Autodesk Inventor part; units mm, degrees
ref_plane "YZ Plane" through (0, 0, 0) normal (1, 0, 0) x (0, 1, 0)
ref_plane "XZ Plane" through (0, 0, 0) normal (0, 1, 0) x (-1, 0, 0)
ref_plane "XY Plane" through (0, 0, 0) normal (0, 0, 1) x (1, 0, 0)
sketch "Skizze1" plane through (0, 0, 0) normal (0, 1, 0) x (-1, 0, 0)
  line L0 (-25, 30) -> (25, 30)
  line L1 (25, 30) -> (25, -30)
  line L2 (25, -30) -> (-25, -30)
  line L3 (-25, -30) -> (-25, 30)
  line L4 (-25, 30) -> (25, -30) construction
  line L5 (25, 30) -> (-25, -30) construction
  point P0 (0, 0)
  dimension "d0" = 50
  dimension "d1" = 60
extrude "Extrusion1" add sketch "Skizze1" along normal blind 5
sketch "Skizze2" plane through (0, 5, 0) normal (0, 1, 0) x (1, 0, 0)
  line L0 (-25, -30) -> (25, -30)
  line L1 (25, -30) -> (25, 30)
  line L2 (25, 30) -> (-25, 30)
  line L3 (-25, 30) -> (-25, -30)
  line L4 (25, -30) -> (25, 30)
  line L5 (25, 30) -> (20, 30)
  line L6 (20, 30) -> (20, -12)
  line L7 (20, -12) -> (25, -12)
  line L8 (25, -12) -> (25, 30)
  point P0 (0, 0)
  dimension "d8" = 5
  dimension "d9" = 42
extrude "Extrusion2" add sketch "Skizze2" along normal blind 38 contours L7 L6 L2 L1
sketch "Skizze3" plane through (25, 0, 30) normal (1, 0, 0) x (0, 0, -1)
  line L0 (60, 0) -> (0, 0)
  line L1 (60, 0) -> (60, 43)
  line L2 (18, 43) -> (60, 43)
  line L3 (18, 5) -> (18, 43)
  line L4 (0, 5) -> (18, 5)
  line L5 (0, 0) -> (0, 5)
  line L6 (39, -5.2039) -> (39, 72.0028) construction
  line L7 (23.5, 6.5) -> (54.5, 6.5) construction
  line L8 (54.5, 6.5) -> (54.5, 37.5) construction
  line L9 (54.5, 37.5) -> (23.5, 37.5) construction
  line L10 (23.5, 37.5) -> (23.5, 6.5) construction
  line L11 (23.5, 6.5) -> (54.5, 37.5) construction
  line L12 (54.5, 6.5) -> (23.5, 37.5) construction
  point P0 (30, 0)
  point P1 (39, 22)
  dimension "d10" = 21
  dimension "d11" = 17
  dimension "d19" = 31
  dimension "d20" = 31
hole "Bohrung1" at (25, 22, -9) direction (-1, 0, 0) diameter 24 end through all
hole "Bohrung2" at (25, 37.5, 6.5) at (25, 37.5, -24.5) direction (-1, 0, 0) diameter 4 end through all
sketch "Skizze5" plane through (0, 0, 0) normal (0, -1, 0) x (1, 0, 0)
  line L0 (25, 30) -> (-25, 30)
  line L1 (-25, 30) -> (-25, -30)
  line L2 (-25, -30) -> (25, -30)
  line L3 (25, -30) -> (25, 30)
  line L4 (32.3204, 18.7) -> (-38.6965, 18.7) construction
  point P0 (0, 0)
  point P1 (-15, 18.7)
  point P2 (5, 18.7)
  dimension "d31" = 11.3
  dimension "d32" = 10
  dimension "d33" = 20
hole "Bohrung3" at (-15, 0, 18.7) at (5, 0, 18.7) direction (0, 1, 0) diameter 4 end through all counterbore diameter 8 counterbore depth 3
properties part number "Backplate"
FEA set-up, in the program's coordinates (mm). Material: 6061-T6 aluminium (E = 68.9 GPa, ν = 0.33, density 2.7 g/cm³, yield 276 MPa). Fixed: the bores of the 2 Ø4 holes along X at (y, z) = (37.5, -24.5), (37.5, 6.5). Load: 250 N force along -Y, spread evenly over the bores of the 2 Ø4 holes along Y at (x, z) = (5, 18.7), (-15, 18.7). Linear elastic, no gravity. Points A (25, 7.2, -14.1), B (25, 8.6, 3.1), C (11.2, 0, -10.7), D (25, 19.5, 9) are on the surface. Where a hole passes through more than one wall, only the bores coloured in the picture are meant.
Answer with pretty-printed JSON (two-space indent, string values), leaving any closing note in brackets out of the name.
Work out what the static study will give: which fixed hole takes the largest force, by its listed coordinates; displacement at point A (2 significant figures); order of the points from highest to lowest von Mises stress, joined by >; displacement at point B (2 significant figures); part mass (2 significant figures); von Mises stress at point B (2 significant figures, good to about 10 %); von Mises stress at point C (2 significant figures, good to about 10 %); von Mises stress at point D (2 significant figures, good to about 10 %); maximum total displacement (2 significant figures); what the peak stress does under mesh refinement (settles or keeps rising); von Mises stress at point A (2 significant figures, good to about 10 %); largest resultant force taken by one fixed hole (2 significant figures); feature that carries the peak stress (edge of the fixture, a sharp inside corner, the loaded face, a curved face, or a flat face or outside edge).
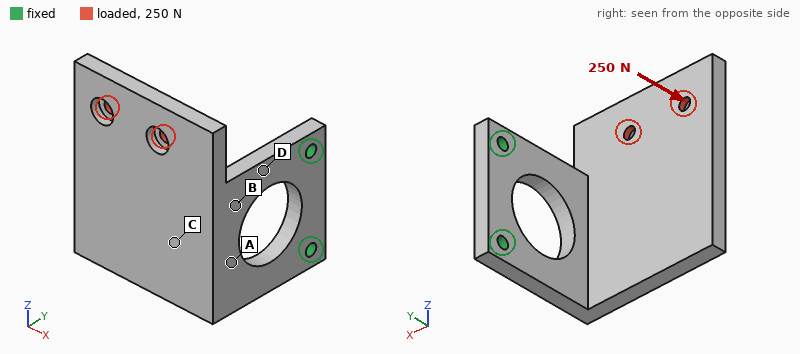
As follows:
{
  "which fixed hole takes the largest force, by its listed coordinates": "(37.5, 6.5)",
  "displacement at point A": "0.19 mm",
  "order of the points from highest to lowest von Mises stress, joined by >": "D > B > A > C",
  "displacement at point B": "0.19 mm",
  "part mass": "55 g",
  "von Mises stress at point B": "51 MPa",
  "von Mises stress at point C": "25 MPa",
  "von Mises stress at point D": "85 MPa",
  "maximum total displacement": "0.94 mm",
  "what the peak stress does under mesh refinement": "keeps rising",
  "von Mises stress at point A": "39 MPa",
  "largest resultant force taken by one fixed hole": "340 N",
  "feature that carries the peak stress": "edge of the fixture"
}
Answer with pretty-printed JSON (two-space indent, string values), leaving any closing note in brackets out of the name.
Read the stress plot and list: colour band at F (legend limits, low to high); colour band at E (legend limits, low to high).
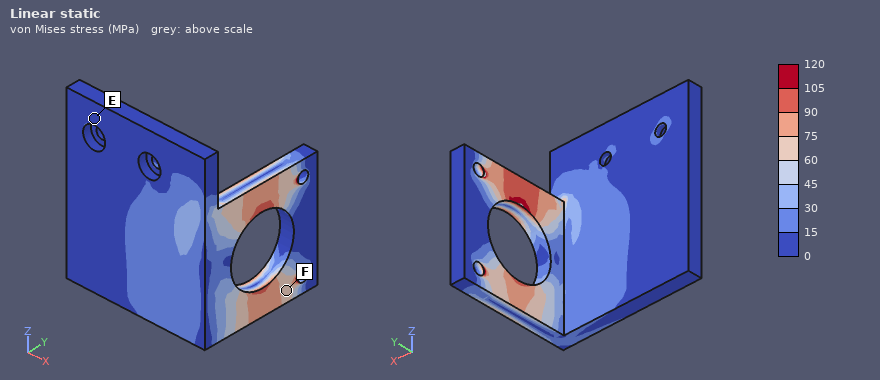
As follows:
{
  "colour band at F": "60 to 75 MPa",
  "colour band at E": "0 to 15 MPa"
}
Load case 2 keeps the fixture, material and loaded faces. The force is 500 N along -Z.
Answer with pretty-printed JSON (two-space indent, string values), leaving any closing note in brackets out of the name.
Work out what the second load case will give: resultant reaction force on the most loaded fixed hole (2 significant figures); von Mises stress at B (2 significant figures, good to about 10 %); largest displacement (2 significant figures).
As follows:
{
  "resultant reaction force on the most loaded fixed hole": "630 N",
  "von Mises stress at B": "57 MPa",
  "largest displacement": "0.58 mm"
}
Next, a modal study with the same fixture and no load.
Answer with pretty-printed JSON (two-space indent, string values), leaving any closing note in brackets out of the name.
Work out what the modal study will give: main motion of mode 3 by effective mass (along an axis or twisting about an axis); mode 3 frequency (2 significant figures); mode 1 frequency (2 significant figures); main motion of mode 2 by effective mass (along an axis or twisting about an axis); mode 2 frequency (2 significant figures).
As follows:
{
  "main motion of mode 3 by effective mass": "along X",
  "mode 3 frequency": "1800 Hz",
  "mode 1 frequency": "510 Hz",
  "main motion of mode 2 by effective mass": "along Z",
  "mode 2 frequency": "950 Hz"
}
